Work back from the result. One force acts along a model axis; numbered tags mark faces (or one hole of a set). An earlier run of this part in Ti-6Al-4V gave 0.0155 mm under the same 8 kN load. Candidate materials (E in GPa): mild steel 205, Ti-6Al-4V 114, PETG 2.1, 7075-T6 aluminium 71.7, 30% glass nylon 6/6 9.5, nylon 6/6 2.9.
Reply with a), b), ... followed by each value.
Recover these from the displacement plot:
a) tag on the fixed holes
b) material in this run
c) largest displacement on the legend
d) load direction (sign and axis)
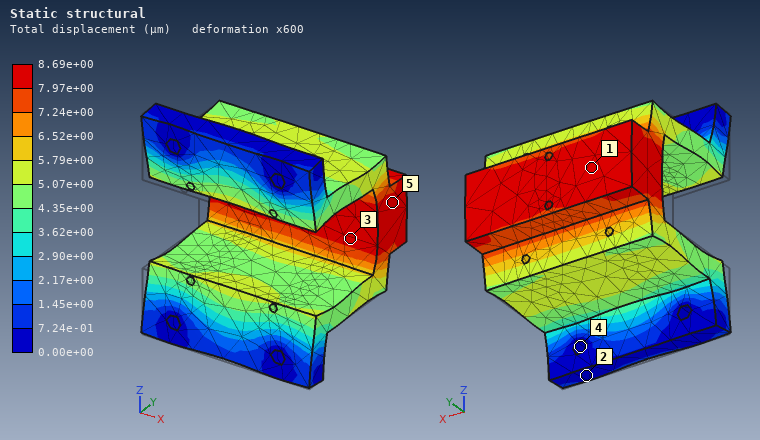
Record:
a) 4
b) mild steel
c) 8.69e+00 µm
d) +Y
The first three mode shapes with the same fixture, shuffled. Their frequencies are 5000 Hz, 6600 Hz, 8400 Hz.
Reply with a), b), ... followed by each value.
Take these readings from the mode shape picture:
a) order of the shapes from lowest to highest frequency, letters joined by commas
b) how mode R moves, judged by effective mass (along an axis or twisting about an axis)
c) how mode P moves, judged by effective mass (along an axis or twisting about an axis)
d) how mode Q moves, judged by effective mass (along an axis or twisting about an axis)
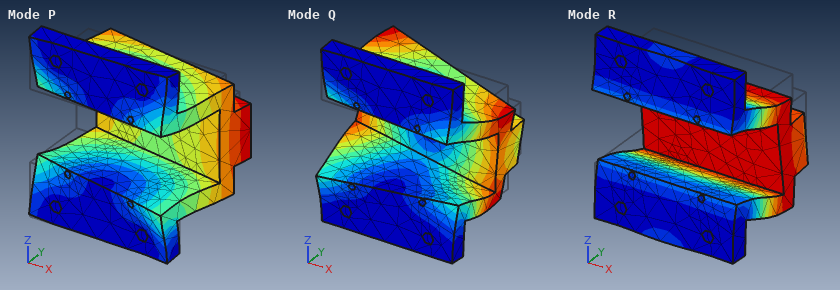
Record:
a) R, P, Q
b) along Z
c) along X
d) twisting about Y
